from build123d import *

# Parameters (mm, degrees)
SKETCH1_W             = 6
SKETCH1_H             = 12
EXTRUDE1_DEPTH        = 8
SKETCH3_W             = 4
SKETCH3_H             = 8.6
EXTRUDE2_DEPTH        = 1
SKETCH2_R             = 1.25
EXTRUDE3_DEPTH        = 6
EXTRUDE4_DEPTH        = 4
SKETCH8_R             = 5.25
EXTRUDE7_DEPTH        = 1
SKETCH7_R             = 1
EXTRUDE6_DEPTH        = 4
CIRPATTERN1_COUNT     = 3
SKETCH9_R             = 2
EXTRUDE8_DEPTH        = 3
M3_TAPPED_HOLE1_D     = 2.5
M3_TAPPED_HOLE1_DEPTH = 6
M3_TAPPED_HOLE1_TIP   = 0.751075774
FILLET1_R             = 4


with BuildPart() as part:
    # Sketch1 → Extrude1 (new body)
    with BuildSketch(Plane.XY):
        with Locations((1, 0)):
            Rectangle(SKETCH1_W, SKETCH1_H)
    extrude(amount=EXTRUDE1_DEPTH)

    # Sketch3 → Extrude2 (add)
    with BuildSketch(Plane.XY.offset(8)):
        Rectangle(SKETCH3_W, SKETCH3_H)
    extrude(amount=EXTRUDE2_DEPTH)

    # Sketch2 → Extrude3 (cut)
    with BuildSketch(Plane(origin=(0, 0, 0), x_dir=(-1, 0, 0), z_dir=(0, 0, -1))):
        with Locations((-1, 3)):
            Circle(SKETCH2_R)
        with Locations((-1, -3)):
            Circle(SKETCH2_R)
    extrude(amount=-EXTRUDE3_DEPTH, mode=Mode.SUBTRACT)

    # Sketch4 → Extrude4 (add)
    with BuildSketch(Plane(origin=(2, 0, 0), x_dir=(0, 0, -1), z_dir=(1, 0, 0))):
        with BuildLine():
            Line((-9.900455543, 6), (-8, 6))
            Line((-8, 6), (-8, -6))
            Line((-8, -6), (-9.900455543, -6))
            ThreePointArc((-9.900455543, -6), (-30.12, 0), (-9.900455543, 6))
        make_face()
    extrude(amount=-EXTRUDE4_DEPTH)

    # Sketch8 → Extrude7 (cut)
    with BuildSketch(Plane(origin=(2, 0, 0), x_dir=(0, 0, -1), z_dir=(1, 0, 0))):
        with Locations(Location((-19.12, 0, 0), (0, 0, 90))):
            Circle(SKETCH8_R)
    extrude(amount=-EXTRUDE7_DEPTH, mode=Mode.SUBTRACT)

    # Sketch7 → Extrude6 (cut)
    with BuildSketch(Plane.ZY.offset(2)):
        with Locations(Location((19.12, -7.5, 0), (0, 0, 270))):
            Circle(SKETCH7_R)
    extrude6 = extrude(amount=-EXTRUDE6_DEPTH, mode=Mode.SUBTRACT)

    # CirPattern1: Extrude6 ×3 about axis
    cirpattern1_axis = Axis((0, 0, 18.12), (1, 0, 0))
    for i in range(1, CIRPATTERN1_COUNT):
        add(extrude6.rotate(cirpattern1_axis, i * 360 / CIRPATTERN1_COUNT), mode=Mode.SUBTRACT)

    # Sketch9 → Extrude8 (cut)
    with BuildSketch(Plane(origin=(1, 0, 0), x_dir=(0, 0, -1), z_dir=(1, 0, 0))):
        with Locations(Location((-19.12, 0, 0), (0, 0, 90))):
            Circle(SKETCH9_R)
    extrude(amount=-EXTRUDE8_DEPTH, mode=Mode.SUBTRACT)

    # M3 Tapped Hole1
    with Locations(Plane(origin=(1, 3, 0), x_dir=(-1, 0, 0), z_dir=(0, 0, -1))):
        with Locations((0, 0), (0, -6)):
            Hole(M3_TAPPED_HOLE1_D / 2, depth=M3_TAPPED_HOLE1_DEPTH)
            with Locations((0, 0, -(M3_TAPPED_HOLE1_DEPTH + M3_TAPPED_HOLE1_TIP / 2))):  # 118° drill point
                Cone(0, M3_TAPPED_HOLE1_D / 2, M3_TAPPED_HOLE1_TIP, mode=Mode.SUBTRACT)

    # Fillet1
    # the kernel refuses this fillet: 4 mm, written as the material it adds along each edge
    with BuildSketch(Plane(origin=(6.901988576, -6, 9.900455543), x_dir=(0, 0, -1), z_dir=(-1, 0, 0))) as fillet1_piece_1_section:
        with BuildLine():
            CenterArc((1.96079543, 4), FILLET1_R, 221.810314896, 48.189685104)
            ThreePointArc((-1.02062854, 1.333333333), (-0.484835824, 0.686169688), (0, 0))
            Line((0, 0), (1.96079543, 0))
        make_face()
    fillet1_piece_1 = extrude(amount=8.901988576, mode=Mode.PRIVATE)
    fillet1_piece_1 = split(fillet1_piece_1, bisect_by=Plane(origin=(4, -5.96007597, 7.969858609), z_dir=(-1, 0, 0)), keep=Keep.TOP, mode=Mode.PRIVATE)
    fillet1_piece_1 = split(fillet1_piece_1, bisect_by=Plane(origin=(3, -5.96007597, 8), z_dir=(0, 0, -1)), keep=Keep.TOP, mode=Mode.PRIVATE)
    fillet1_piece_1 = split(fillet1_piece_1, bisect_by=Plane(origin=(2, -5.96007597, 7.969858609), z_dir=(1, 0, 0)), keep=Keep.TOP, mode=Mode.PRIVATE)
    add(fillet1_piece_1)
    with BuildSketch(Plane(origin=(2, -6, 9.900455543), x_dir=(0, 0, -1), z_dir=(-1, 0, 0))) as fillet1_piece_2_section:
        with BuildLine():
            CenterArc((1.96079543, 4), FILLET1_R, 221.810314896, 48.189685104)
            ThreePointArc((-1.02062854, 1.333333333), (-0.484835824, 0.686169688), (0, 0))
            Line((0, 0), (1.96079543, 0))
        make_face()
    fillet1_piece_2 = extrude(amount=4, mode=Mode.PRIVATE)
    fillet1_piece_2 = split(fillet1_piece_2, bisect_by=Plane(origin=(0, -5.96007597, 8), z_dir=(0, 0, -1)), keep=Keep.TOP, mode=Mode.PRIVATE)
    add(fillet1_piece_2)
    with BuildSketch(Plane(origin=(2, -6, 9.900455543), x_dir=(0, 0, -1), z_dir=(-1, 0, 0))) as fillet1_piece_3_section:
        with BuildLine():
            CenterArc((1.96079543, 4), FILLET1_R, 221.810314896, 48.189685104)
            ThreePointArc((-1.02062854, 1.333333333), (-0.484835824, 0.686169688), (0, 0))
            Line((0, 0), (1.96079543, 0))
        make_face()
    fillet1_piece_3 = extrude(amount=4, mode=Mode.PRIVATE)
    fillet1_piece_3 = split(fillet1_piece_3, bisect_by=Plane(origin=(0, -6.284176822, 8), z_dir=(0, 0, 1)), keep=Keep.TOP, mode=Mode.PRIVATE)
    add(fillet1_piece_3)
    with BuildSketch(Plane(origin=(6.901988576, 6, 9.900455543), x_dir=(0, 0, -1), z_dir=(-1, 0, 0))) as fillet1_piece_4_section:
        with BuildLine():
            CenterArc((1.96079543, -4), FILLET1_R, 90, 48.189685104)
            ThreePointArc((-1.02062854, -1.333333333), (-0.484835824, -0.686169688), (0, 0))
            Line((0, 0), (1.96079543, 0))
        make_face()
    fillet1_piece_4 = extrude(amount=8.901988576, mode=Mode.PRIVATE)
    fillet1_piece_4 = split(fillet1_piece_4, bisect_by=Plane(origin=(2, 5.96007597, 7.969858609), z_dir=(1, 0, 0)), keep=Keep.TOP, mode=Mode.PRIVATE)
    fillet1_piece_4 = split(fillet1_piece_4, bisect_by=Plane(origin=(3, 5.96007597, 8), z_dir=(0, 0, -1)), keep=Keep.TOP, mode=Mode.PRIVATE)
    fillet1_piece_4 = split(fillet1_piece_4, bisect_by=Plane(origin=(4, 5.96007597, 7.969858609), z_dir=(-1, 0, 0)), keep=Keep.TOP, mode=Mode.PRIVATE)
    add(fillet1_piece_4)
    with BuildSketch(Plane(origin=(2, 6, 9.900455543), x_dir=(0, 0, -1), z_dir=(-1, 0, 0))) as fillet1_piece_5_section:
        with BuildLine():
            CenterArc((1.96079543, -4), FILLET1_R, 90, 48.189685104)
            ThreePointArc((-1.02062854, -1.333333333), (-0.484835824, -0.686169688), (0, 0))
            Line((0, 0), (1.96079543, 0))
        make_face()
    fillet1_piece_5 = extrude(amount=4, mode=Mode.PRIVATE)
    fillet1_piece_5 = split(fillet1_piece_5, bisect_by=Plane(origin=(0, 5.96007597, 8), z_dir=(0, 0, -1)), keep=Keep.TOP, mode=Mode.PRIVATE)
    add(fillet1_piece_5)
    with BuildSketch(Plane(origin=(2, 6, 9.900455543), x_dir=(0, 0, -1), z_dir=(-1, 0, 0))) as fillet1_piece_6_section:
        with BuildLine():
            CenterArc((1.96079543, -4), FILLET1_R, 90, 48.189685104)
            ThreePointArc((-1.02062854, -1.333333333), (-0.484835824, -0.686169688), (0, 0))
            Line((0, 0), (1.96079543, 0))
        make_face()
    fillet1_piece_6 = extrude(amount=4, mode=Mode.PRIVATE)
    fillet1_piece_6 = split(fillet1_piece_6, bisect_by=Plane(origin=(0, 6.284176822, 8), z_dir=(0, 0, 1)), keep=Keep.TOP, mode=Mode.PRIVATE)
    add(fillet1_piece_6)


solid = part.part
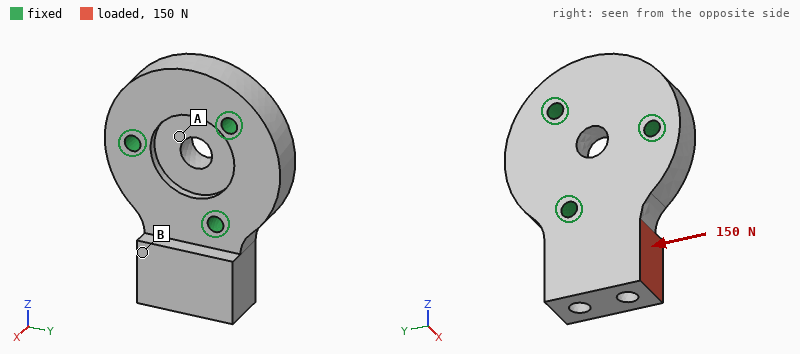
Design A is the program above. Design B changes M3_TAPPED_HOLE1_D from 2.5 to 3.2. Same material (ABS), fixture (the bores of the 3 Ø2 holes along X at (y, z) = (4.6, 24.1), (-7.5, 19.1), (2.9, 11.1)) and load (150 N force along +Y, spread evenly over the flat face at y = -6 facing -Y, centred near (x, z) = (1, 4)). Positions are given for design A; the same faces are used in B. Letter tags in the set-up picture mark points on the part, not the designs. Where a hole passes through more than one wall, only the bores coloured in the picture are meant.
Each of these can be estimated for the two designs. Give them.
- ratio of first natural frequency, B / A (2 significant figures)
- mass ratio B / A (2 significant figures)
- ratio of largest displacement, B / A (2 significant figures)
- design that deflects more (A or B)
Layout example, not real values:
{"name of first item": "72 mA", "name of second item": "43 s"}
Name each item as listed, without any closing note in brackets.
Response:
{"ratio of first natural frequency, B / A": "1.0", "mass ratio B / A": "0.98", "ratio of largest displacement, B / A": "1.1", "design that deflects more": "B"}
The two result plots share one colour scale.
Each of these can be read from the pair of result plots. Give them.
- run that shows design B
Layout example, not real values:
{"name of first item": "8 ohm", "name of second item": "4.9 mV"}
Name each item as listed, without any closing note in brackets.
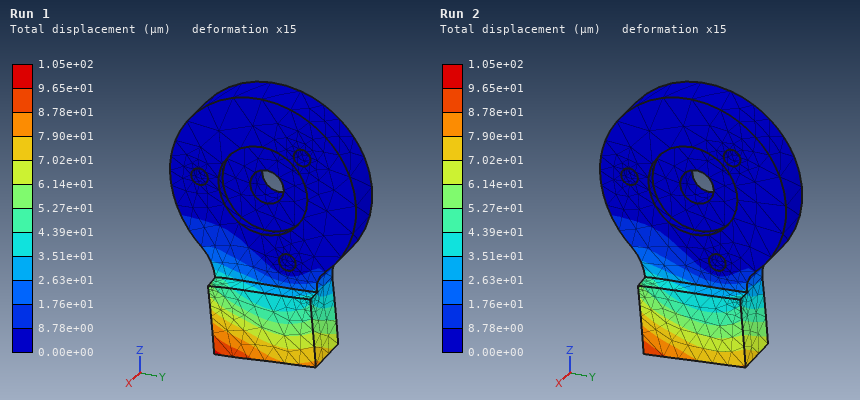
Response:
{"run that shows design B": "Run 1"}
